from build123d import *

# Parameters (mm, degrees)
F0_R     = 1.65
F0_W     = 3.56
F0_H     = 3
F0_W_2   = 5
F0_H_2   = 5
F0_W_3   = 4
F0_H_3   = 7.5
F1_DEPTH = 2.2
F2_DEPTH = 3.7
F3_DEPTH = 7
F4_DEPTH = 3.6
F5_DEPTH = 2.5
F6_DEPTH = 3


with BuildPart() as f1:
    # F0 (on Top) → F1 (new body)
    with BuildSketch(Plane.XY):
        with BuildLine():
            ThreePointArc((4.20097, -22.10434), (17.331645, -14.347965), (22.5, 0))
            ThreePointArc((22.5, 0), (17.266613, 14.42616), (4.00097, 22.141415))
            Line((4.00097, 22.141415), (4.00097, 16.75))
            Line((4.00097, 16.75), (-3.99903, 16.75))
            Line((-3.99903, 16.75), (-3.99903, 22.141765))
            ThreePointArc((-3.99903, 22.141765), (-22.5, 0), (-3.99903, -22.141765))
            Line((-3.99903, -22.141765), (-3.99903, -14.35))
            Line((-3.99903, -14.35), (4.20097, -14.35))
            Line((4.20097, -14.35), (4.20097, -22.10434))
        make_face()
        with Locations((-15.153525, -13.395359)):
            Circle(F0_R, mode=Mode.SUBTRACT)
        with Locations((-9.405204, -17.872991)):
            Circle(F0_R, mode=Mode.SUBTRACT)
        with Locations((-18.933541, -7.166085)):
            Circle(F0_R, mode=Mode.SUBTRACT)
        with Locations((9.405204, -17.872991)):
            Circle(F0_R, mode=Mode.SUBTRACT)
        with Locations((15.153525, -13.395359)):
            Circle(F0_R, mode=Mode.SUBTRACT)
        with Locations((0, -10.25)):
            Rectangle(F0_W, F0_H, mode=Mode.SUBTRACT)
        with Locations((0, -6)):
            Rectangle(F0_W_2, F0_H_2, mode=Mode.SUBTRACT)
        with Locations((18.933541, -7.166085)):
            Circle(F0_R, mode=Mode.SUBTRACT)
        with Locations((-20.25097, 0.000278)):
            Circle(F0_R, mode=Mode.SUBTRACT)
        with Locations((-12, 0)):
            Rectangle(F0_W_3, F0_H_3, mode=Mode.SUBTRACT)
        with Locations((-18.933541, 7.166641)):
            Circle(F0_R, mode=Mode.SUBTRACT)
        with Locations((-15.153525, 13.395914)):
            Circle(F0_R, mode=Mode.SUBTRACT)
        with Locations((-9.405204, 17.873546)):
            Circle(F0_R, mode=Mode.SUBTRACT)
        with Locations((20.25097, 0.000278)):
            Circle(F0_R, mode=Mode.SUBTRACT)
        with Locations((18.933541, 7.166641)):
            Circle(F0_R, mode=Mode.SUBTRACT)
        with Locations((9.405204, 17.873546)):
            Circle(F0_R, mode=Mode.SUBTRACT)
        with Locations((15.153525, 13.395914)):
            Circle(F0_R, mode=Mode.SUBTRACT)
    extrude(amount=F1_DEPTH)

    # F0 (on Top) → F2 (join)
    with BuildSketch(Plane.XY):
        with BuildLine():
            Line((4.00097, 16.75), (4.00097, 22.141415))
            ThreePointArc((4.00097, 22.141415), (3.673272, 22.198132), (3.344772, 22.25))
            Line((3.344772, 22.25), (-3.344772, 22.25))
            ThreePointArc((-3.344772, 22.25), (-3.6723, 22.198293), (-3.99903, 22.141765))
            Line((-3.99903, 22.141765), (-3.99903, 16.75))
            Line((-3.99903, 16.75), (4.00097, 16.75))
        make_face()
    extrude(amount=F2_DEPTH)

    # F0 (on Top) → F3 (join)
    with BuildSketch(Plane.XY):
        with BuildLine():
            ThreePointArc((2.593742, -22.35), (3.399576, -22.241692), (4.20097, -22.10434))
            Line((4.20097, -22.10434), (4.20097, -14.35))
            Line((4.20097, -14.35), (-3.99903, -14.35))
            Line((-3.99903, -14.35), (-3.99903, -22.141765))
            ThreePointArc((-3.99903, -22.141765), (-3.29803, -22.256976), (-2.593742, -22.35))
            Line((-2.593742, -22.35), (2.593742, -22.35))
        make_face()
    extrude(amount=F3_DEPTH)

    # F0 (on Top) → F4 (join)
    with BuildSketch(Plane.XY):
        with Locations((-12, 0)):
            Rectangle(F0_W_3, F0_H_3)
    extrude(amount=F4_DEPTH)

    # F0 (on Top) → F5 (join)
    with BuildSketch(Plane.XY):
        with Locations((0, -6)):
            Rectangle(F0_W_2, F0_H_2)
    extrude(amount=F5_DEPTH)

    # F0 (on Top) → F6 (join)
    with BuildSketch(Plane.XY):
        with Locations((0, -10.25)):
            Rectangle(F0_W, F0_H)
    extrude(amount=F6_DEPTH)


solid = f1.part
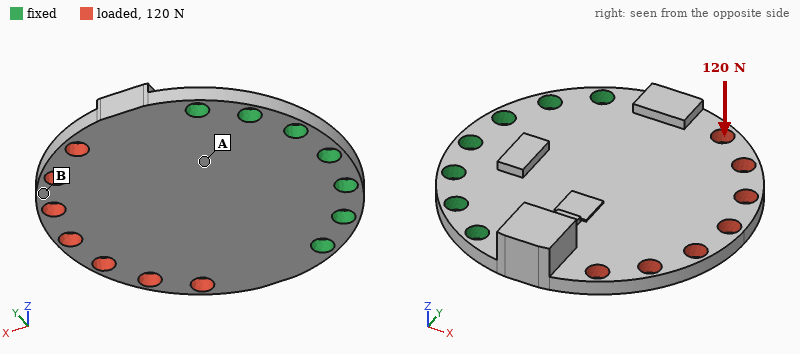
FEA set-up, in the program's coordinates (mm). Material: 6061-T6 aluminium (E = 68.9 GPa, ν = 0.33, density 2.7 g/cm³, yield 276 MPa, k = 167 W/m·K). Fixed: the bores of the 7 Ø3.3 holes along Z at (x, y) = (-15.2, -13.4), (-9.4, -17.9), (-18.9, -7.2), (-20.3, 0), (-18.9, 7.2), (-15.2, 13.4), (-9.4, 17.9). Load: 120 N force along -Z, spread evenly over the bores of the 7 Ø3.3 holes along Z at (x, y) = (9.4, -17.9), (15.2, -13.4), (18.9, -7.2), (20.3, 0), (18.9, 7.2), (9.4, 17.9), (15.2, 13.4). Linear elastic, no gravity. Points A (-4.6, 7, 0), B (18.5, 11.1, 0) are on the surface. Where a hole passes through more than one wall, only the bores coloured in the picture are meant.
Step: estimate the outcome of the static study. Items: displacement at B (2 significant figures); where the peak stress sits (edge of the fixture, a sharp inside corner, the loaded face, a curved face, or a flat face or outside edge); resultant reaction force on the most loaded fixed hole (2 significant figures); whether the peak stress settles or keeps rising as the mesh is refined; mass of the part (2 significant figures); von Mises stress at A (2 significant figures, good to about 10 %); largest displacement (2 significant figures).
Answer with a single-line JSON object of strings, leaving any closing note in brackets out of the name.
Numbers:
{"displacement at B": "0.27 mm", "where the peak stress sits": "edge of the fixture", "resultant reaction force on the most loaded fixed hole": "110 N", "whether the peak stress settles or keeps rising as the mesh is refined": "keeps rising", "mass of the part": "9.9 g", "von Mises stress at A": "46 MPa", "largest displacement": "0.34 mm"}
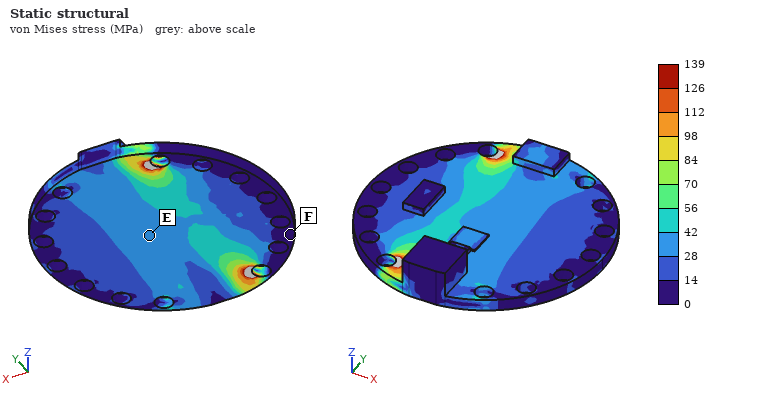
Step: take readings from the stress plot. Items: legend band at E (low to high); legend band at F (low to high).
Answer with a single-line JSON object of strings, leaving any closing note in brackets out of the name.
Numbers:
{"legend band at E": "28 to 42 MPa", "legend band at F": "0 to 14 MPa"}
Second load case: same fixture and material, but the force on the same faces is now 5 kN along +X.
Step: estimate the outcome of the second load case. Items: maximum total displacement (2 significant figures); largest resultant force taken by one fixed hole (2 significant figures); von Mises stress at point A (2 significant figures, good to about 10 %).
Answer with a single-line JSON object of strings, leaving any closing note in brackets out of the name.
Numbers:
{"maximum total displacement": "41 µm", "largest resultant force taken by one fixed hole": "1.3 kN", "von Mises stress at point A": "44 MPa"}
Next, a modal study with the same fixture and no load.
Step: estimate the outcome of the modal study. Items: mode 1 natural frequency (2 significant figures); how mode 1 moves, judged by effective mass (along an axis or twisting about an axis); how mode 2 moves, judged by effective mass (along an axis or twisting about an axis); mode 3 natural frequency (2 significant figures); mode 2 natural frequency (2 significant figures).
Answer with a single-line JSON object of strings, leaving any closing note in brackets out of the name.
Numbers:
{"mode 1 natural frequency": "2300 Hz", "how mode 1 moves, judged by effective mass": "along Z", "how mode 2 moves, judged by effective mass": "twisting about X", "mode 3 natural frequency": "9700 Hz", "mode 2 natural frequency": "5400 Hz"}
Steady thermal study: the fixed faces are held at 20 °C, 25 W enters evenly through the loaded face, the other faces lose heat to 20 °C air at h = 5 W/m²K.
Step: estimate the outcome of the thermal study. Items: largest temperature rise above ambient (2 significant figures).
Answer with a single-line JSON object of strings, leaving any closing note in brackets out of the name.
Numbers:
{"largest temperature rise above ambient": "49 K"}
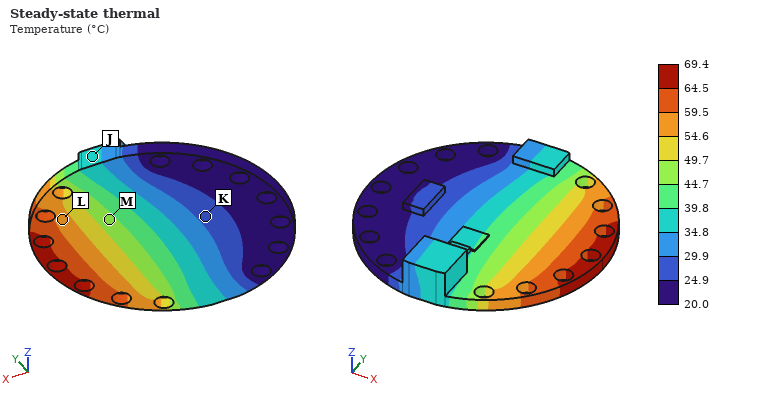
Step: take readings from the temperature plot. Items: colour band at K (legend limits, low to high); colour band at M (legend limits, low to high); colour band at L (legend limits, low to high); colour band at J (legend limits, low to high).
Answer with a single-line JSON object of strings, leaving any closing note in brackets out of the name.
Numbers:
{"colour band at K": "24.9 to 29.9 °C", "colour band at M": "44.7 to 49.7 °C", "colour band at L": "54.6 to 59.5 °C", "colour band at J": "34.8 to 39.8 °C"}
